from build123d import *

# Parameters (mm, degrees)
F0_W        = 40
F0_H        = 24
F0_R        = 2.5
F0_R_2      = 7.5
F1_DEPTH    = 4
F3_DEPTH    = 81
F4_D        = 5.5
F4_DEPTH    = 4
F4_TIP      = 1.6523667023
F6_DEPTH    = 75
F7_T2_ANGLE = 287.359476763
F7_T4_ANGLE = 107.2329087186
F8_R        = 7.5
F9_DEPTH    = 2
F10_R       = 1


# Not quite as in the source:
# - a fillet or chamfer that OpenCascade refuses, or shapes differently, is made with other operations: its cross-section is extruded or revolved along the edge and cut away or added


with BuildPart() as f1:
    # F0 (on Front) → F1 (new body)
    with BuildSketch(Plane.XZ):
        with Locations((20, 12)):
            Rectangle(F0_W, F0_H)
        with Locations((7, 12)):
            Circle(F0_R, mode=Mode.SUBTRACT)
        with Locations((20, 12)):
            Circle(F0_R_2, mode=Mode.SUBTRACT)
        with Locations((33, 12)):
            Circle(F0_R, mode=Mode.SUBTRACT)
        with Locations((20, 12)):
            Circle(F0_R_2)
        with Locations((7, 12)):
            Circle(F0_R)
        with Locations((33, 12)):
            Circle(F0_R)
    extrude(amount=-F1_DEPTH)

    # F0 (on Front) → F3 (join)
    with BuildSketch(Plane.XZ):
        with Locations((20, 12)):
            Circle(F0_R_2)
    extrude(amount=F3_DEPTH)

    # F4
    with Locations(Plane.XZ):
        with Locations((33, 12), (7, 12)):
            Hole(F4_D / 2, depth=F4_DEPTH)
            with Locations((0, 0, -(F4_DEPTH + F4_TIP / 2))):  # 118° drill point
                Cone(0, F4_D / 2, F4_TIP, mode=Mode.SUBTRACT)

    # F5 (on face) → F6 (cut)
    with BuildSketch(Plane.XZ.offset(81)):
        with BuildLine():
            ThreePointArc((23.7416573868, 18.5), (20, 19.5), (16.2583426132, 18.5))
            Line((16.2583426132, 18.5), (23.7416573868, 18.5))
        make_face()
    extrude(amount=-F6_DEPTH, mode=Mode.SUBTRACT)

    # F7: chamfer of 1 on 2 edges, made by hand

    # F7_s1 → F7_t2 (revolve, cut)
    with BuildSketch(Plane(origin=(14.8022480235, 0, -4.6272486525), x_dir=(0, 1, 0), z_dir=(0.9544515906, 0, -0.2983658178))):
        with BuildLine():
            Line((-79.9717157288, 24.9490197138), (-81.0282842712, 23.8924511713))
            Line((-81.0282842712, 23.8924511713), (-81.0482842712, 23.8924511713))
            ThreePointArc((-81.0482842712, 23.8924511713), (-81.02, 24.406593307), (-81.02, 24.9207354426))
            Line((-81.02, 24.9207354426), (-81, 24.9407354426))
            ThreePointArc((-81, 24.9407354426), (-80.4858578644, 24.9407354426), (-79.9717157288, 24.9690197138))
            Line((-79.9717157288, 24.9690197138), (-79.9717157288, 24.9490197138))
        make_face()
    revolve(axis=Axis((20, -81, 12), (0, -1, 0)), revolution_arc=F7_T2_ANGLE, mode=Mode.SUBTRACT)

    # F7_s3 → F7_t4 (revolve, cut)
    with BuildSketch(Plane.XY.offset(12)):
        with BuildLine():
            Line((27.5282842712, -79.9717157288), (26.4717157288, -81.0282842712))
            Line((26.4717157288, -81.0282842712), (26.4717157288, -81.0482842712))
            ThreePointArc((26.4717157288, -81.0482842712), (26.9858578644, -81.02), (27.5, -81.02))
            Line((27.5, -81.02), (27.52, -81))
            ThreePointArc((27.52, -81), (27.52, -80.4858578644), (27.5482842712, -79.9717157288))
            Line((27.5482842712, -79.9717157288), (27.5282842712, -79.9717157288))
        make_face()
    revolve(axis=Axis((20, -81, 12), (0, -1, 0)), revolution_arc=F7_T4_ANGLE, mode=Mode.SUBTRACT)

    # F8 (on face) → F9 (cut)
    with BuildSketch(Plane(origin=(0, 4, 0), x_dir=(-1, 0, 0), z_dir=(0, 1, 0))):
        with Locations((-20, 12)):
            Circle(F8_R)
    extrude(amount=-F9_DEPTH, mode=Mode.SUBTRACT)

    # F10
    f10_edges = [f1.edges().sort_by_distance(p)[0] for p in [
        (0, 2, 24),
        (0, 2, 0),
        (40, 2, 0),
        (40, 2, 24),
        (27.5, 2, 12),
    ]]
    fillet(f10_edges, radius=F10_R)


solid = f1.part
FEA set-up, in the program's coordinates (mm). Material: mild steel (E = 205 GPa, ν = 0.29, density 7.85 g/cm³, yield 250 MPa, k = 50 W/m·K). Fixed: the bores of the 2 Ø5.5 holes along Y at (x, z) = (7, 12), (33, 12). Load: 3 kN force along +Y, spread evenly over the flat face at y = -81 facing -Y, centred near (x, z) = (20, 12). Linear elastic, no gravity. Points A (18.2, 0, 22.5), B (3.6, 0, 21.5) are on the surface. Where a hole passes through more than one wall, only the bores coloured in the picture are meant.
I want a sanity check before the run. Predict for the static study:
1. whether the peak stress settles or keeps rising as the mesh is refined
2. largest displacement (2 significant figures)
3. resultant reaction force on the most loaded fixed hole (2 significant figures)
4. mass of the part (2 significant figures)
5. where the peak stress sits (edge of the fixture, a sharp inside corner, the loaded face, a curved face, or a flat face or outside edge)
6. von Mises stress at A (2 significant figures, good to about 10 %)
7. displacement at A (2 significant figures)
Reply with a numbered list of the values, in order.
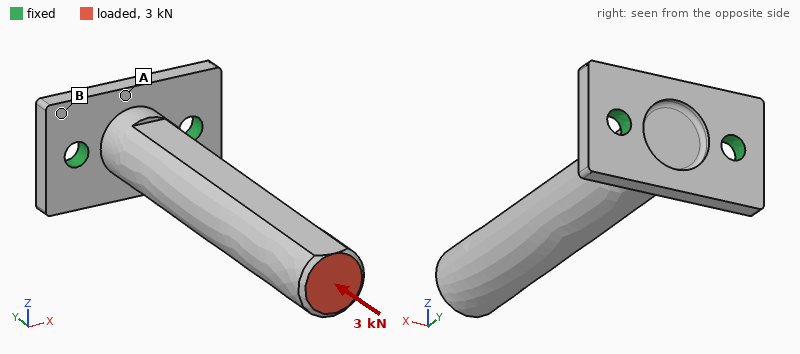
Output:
1. keeps rising
2. 13 µm
3. 1.7 kN
4. 140 g
5. edge of the fixture
6. 25 MPa
7. 5.5 µm
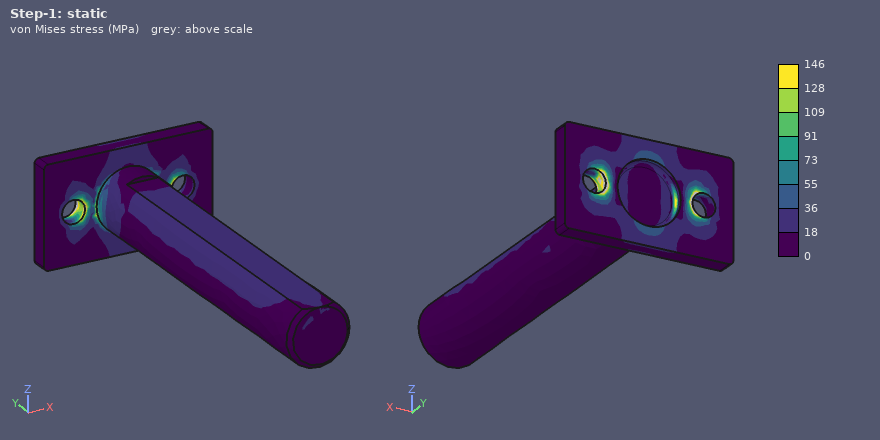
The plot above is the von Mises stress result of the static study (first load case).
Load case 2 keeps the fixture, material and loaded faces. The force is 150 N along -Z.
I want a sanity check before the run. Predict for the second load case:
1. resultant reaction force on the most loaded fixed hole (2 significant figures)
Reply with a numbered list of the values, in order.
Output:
1. 75 N
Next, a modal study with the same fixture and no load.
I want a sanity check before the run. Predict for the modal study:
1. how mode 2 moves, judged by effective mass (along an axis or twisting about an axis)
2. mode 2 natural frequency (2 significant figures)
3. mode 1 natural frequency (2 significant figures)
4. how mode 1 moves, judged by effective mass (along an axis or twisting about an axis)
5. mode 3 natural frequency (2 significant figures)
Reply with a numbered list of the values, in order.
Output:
1. along X
2. 1300 Hz
3. 840 Hz
4. along Z
5. 6700 Hz
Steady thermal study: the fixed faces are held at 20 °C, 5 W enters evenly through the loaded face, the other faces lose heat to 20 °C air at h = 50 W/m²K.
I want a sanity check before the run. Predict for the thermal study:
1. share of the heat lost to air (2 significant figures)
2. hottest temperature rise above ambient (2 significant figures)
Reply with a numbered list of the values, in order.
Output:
1. 60 %
2. 32 K
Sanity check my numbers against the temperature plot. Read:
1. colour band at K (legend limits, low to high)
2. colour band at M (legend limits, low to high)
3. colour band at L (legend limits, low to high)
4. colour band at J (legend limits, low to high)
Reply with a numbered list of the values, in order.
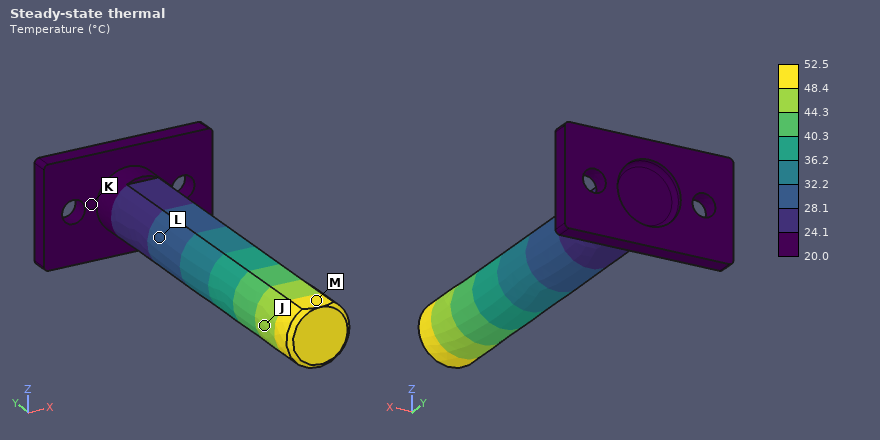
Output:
1. 20.0 to 24.1 °C
2. 48.4 to 52.5 °C
3. 28.1 to 32.2 °C
4. 44.3 to 48.4 °C
